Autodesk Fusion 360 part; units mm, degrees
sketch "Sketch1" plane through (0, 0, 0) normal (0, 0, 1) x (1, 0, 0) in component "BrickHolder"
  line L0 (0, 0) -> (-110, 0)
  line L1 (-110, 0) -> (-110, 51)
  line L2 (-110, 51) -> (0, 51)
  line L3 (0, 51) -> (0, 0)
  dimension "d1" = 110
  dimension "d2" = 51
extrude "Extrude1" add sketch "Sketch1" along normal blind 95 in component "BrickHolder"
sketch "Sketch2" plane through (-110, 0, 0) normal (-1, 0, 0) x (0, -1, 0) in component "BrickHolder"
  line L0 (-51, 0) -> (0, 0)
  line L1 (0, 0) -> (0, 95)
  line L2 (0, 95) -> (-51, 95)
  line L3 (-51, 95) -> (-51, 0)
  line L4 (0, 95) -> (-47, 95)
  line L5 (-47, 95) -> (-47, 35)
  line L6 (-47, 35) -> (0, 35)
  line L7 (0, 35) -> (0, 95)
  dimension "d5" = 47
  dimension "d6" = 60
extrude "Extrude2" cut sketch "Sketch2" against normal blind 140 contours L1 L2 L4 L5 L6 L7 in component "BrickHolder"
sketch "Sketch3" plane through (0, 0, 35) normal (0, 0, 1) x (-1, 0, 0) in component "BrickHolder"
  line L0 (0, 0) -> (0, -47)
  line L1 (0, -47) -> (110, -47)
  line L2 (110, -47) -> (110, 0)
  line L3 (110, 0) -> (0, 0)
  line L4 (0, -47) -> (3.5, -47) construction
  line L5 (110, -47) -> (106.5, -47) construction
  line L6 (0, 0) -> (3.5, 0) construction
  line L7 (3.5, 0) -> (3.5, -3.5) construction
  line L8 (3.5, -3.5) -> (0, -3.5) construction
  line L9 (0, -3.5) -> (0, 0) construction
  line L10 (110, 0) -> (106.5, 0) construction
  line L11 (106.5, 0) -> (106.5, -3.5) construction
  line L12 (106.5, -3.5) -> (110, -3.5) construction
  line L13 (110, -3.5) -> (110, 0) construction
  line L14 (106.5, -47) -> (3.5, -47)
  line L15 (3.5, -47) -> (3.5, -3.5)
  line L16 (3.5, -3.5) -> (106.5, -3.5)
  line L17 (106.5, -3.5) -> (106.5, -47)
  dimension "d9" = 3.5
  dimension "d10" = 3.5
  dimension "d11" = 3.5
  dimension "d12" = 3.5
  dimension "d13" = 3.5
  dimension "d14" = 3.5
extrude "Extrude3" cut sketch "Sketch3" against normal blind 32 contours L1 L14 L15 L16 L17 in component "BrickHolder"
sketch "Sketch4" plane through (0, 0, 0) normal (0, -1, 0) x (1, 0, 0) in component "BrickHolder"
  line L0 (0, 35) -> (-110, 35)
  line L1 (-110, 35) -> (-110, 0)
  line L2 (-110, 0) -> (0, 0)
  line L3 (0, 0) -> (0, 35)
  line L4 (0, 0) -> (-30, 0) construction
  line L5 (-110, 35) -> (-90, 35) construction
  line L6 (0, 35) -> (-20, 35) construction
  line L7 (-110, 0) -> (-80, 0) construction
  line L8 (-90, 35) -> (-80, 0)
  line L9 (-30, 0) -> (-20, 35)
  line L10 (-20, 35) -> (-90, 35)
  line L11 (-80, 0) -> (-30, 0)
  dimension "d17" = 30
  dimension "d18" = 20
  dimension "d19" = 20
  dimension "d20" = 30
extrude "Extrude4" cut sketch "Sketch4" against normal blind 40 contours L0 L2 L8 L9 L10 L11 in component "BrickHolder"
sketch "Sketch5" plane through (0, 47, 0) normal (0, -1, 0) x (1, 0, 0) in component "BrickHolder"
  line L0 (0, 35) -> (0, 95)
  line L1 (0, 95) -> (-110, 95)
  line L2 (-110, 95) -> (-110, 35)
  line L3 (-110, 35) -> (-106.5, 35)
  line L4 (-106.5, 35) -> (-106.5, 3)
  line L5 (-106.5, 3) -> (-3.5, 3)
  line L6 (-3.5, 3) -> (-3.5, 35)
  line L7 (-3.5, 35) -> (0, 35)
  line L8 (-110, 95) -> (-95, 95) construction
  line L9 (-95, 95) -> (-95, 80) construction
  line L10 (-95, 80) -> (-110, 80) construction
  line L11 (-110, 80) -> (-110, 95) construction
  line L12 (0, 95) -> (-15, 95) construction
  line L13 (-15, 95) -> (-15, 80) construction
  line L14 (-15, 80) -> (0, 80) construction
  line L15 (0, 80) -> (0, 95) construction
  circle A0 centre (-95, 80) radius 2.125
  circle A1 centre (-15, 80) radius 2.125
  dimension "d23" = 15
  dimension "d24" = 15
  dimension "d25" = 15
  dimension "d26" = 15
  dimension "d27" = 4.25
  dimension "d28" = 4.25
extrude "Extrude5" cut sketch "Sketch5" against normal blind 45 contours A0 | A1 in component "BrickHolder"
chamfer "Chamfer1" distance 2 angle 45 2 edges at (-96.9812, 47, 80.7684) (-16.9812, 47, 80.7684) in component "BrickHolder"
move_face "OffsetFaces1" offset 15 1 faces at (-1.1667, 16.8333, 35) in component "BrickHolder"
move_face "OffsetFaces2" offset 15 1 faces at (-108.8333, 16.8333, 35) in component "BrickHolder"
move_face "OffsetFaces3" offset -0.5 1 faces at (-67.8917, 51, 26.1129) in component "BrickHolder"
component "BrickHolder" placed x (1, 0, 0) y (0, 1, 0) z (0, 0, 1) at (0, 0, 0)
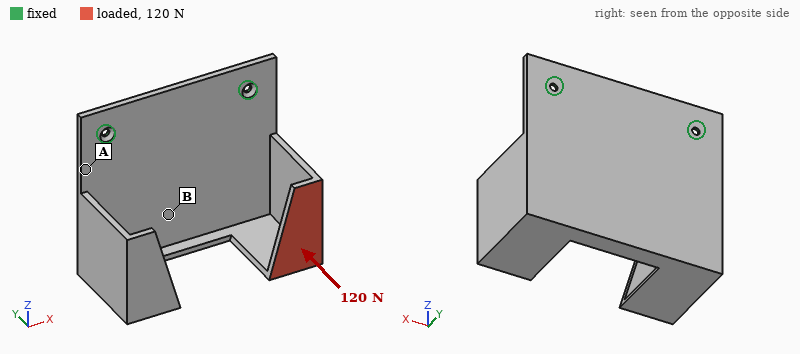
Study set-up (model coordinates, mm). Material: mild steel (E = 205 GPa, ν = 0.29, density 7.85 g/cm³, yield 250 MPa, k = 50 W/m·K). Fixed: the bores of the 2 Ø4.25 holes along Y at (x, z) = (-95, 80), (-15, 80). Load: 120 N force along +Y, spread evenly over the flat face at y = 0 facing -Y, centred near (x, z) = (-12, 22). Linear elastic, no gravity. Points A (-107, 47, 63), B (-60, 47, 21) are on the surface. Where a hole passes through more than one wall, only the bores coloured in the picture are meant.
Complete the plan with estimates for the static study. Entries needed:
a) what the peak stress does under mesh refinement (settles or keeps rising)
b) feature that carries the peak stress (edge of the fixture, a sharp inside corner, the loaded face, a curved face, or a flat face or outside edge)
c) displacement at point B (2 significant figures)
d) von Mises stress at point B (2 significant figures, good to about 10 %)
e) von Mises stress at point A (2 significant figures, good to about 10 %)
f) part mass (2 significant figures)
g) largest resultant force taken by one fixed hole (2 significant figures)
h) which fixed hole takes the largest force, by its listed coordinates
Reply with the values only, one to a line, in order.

keeps rising
edge of the fixture
0.18 mm
9.1 MPa
28 MPa
530 g
120 N
(-15, 80)
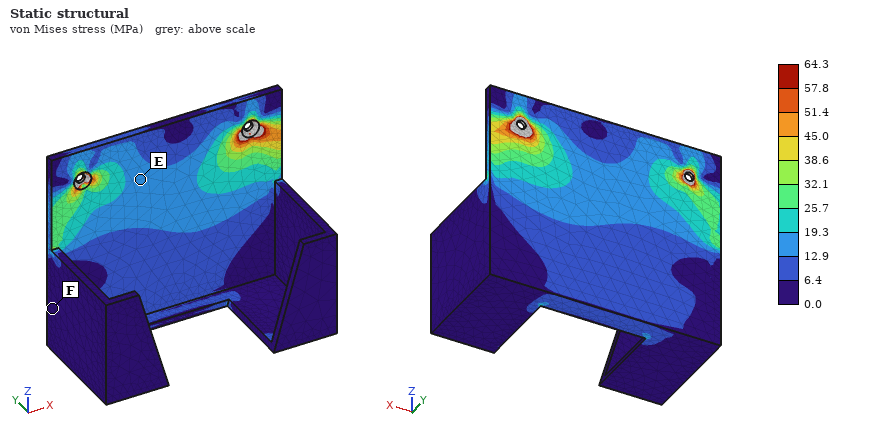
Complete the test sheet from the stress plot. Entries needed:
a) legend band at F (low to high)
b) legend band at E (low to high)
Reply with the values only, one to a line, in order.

0.0 to 6.4 MPa
12.9 to 19.3 MPa
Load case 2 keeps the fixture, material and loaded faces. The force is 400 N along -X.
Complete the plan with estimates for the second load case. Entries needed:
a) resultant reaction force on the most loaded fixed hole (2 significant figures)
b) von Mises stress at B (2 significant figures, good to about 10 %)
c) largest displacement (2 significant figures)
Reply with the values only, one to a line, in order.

440 N
47 MPa
0.63 mm
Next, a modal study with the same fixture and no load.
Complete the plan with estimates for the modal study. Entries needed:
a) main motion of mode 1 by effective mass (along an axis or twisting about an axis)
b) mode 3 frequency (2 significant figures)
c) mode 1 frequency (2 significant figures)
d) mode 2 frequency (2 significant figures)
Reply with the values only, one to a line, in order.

along Y
820 Hz
170 Hz
300 Hz
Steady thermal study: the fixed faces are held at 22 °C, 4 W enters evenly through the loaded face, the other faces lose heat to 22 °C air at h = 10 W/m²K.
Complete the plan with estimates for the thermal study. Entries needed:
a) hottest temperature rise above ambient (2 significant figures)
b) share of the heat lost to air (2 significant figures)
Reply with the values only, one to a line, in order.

25 K
63 %
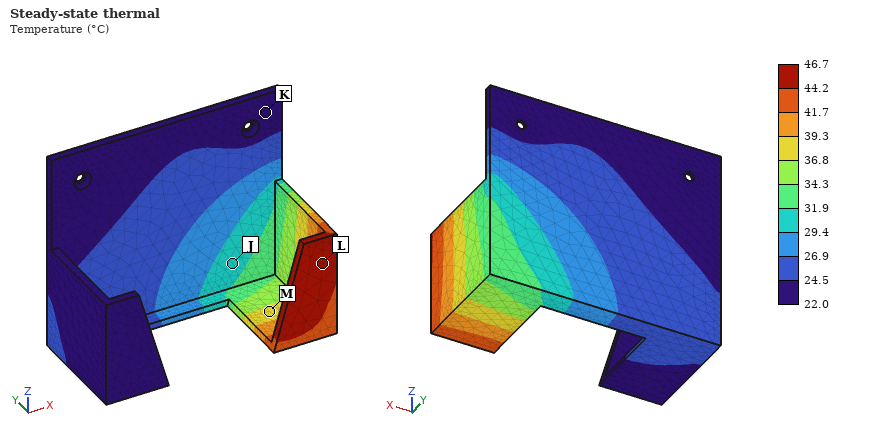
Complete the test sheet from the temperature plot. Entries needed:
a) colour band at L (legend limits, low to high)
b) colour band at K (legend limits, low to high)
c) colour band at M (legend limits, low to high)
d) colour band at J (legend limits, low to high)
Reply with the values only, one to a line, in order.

44.2 to 46.7 °C
22.0 to 24.5 °C
36.8 to 39.3 °C
29.4 to 31.9 °C
